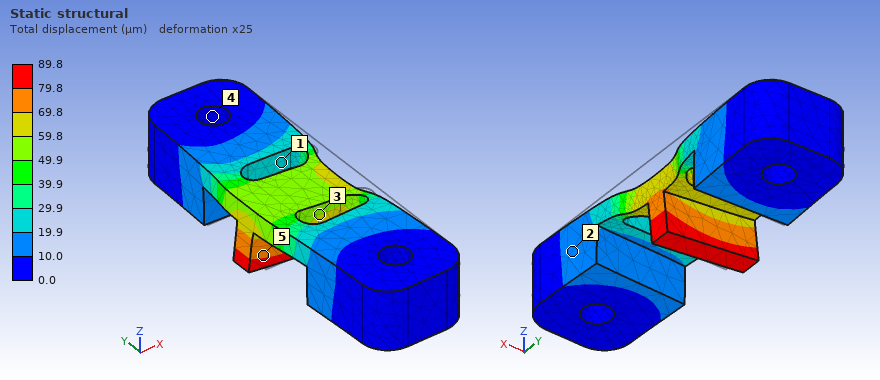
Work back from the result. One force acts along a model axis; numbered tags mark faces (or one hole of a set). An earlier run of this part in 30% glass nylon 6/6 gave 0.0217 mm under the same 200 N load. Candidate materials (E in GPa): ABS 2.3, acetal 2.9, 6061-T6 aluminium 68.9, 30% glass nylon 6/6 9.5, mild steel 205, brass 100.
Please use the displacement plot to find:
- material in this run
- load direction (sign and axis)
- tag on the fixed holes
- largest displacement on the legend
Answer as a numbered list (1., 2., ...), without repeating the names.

1. ABS
2. -X
3. 4
4. 89.8 µm
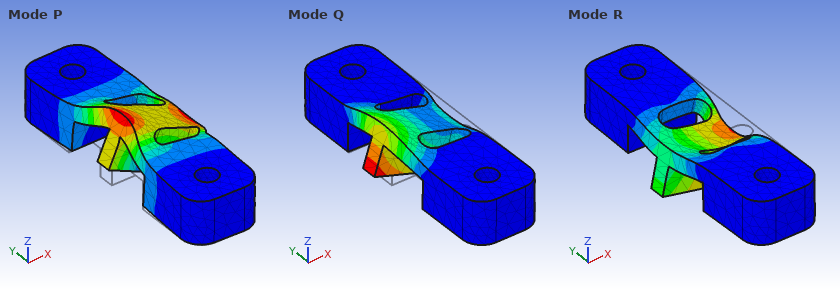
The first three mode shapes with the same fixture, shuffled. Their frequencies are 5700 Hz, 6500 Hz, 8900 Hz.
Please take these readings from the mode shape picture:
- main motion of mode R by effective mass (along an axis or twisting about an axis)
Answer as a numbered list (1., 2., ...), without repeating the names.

1. along Z
